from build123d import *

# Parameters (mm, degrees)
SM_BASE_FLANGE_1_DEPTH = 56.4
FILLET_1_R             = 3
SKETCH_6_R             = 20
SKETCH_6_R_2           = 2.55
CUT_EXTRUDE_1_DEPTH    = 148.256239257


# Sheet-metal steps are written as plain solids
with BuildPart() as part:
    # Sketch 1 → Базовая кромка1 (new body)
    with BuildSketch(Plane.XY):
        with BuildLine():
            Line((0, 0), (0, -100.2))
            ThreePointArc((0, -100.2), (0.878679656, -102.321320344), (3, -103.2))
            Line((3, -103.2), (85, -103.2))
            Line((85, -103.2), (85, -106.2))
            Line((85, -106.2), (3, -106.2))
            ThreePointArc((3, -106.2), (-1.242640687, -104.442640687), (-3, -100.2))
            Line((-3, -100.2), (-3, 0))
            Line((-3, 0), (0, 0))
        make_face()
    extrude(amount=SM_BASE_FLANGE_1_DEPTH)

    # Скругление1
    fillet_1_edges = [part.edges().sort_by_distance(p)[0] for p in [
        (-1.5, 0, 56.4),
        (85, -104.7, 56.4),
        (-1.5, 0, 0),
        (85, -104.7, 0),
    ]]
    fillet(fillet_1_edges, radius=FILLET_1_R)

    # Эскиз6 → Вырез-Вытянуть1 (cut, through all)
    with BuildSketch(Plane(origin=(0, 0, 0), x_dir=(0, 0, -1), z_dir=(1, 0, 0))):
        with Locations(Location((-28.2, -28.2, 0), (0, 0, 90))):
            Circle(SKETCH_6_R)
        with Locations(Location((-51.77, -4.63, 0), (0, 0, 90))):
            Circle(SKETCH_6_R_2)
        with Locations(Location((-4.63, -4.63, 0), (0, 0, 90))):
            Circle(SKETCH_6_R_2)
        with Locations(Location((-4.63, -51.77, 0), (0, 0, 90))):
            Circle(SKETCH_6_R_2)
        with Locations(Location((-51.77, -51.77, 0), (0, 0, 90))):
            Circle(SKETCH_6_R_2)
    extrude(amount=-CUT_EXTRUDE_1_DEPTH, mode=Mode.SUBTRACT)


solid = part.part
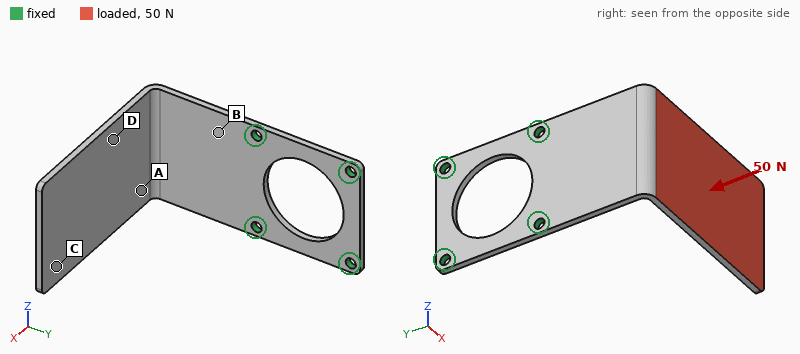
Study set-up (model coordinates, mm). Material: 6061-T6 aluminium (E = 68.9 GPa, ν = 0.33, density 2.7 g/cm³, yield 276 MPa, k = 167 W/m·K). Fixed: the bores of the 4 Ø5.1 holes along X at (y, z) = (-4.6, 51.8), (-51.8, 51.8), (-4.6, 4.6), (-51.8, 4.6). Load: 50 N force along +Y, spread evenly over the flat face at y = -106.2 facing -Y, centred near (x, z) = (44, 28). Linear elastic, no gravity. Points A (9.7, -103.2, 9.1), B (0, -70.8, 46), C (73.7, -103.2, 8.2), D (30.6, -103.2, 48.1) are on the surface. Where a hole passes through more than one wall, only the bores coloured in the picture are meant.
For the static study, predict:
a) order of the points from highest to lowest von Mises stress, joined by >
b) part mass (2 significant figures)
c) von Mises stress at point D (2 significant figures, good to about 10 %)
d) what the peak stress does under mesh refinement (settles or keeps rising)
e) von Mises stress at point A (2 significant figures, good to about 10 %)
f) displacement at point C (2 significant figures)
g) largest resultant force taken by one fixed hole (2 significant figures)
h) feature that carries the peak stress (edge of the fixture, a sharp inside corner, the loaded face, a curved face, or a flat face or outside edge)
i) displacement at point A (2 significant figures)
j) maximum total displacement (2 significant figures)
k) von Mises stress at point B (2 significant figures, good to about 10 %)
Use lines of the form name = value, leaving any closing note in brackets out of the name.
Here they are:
order of the points from highest to lowest von Mises stress, joined by > = B > A > D > C
part mass = 76 g
von Mises stress at point D = 10 MPa
what the peak stress does under mesh refinement = keeps rising
von Mises stress at point A = 18 MPa
displacement at point C = 1.4 mm
largest resultant force taken by one fixed hole = 26 N
feature that carries the peak stress = edge of the fixture
displacement at point A = 0.40 mm
maximum total displacement = 1.7 mm
von Mises stress at point B = 26 MPa
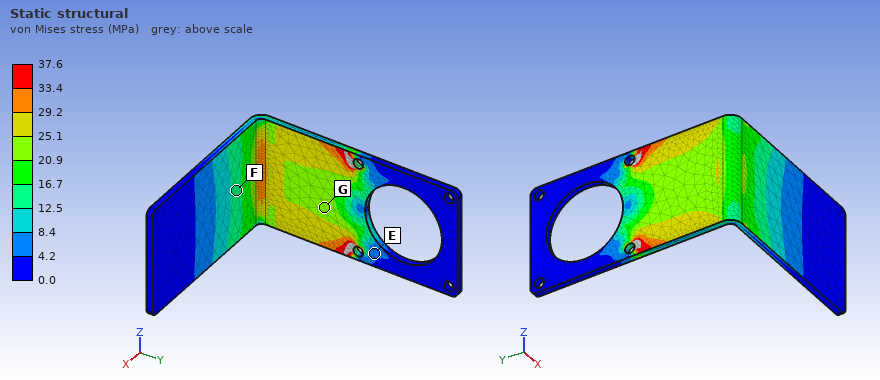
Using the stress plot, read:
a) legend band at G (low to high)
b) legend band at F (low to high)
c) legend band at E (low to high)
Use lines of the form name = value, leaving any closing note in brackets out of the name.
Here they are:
legend band at G = 20.9 to 25.1 MPa
legend band at F = 12.5 to 16.7 MPa
legend band at E = 4.2 to 8.4 MPa
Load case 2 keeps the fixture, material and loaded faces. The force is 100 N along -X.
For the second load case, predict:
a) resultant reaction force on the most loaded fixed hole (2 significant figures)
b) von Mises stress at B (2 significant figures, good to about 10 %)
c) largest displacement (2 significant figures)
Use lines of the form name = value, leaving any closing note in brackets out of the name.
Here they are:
resultant reaction force on the most loaded fixed hole = 55 N
von Mises stress at B = 41 MPa
largest displacement = 1.7 mm
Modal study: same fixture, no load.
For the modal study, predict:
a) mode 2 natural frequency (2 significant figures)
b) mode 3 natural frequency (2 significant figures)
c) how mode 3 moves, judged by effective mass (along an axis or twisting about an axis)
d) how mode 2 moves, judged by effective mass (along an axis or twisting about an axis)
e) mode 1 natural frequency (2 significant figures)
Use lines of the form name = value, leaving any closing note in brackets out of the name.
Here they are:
mode 2 natural frequency = 300 Hz
mode 3 natural frequency = 500 Hz
how mode 3 moves, judged by effective mass = along X
how mode 2 moves, judged by effective mass = along Z
mode 1 natural frequency = 160 Hz
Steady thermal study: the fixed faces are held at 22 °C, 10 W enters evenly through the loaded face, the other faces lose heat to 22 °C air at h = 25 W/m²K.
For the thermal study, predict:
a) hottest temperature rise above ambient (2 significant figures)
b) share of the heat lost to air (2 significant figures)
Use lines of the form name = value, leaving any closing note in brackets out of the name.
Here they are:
hottest temperature rise above ambient = 24 K
share of the heat lost to air = 40 %
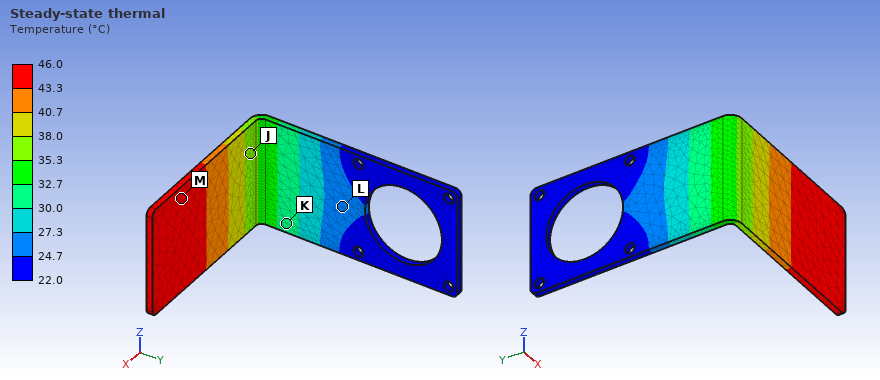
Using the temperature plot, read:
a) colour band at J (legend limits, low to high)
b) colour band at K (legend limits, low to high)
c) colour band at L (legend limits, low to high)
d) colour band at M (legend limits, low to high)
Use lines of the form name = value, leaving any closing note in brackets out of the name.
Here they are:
colour band at J = 35.3 to 38.0 °C
colour band at K = 30.0 to 32.7 °C
colour band at L = 24.7 to 27.3 °C
colour band at M = 43.3 to 46.0 °C
